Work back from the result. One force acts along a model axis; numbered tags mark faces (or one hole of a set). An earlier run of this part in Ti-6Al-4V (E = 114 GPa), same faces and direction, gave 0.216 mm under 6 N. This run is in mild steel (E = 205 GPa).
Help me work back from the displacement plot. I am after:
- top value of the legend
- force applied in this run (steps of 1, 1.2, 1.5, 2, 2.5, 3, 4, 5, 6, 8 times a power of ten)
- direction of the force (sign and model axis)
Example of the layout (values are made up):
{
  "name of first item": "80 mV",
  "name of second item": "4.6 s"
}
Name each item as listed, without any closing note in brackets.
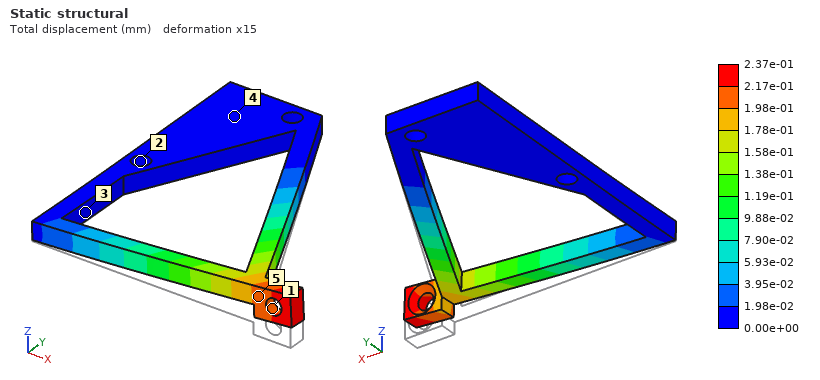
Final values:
{
  "top value of the legend": "2.37e-01 mm",
  "force applied in this run": "12 N",
  "direction of the force": "+Z"
}
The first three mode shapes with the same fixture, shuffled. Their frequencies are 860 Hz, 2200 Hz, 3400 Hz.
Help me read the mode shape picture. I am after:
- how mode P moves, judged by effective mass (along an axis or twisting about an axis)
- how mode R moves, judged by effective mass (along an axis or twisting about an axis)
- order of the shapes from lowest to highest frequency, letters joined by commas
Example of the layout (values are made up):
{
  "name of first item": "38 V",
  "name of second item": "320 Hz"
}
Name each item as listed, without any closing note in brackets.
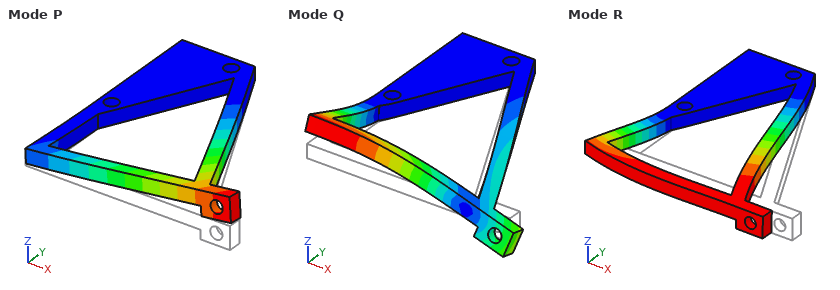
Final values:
{
  "how mode P moves, judged by effective mass": "along Z",
  "how mode R moves, judged by effective mass": "along X",
  "order of the shapes from lowest to highest frequency, letters joined by commas": "P, R, Q"
}
